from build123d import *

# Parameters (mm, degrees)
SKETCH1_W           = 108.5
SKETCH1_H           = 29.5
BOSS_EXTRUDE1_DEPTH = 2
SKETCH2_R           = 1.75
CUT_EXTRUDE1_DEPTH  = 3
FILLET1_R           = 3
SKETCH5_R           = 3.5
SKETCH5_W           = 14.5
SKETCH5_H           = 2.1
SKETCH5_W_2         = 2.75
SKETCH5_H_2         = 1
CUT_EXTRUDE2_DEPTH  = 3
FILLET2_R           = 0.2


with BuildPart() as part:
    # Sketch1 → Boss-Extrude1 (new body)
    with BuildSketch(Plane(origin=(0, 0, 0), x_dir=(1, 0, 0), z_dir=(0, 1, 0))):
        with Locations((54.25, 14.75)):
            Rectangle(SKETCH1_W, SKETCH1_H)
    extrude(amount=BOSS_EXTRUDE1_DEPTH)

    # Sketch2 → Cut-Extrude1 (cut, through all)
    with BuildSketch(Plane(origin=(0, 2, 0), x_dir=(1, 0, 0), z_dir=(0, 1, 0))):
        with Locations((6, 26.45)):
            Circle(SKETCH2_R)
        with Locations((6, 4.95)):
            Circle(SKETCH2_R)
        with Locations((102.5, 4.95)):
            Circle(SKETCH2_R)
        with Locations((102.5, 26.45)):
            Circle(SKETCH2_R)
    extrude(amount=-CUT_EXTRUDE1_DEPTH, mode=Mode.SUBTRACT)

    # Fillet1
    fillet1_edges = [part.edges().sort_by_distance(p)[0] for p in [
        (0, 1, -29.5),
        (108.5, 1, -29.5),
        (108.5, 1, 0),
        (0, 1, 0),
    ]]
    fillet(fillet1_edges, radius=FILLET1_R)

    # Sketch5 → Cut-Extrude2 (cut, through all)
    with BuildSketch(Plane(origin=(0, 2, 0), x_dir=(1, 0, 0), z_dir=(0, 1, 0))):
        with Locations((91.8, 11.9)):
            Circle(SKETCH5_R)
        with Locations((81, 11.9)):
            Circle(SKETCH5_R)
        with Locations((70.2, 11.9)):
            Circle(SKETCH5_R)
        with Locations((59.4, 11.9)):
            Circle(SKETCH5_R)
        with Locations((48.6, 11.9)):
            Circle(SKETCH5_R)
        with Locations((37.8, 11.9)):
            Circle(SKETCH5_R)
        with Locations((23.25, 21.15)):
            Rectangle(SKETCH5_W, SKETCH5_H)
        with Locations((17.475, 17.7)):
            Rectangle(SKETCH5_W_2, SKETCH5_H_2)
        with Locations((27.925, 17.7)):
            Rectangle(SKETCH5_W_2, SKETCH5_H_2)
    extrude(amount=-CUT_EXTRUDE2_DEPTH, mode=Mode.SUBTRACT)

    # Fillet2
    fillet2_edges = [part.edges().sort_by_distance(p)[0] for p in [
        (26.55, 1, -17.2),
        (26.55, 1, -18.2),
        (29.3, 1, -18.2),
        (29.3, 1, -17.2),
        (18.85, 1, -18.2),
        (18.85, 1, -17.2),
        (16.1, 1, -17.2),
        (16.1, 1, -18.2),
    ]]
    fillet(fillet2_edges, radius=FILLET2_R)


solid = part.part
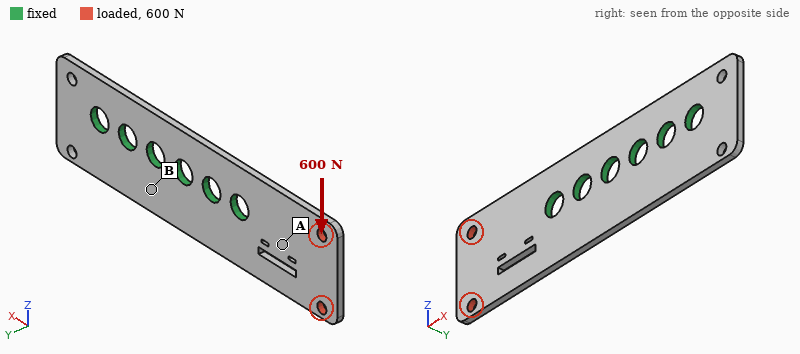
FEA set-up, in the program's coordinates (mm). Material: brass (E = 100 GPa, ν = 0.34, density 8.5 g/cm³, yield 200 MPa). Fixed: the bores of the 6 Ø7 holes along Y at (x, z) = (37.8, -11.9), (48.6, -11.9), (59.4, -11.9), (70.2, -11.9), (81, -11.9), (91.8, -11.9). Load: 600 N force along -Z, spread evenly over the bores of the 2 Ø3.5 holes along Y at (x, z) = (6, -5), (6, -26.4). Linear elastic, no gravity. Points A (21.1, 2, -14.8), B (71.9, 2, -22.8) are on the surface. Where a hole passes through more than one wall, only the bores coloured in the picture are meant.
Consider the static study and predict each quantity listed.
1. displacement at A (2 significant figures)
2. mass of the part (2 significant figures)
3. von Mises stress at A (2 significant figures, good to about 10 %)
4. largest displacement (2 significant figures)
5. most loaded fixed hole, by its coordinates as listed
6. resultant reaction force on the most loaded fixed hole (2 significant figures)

20 µm
49 g
27 MPa
53 µm
(37.8, -11.9)
1.1 kN
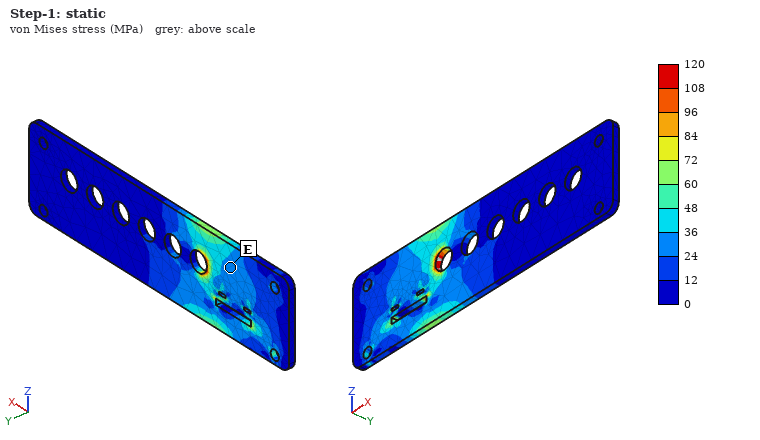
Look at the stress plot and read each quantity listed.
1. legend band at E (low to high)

24 to 36 MPa
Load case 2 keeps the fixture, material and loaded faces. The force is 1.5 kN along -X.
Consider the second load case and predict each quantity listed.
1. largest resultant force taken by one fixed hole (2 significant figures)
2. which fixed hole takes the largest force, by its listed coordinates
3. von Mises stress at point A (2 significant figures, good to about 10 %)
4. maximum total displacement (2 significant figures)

1.0 kN
(37.8, -11.9)
27 MPa
20 µm
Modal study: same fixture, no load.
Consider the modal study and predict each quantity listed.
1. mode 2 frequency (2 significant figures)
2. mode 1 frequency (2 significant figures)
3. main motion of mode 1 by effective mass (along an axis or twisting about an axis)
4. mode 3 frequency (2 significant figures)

2100 Hz
860 Hz
along Y
4100 Hz
